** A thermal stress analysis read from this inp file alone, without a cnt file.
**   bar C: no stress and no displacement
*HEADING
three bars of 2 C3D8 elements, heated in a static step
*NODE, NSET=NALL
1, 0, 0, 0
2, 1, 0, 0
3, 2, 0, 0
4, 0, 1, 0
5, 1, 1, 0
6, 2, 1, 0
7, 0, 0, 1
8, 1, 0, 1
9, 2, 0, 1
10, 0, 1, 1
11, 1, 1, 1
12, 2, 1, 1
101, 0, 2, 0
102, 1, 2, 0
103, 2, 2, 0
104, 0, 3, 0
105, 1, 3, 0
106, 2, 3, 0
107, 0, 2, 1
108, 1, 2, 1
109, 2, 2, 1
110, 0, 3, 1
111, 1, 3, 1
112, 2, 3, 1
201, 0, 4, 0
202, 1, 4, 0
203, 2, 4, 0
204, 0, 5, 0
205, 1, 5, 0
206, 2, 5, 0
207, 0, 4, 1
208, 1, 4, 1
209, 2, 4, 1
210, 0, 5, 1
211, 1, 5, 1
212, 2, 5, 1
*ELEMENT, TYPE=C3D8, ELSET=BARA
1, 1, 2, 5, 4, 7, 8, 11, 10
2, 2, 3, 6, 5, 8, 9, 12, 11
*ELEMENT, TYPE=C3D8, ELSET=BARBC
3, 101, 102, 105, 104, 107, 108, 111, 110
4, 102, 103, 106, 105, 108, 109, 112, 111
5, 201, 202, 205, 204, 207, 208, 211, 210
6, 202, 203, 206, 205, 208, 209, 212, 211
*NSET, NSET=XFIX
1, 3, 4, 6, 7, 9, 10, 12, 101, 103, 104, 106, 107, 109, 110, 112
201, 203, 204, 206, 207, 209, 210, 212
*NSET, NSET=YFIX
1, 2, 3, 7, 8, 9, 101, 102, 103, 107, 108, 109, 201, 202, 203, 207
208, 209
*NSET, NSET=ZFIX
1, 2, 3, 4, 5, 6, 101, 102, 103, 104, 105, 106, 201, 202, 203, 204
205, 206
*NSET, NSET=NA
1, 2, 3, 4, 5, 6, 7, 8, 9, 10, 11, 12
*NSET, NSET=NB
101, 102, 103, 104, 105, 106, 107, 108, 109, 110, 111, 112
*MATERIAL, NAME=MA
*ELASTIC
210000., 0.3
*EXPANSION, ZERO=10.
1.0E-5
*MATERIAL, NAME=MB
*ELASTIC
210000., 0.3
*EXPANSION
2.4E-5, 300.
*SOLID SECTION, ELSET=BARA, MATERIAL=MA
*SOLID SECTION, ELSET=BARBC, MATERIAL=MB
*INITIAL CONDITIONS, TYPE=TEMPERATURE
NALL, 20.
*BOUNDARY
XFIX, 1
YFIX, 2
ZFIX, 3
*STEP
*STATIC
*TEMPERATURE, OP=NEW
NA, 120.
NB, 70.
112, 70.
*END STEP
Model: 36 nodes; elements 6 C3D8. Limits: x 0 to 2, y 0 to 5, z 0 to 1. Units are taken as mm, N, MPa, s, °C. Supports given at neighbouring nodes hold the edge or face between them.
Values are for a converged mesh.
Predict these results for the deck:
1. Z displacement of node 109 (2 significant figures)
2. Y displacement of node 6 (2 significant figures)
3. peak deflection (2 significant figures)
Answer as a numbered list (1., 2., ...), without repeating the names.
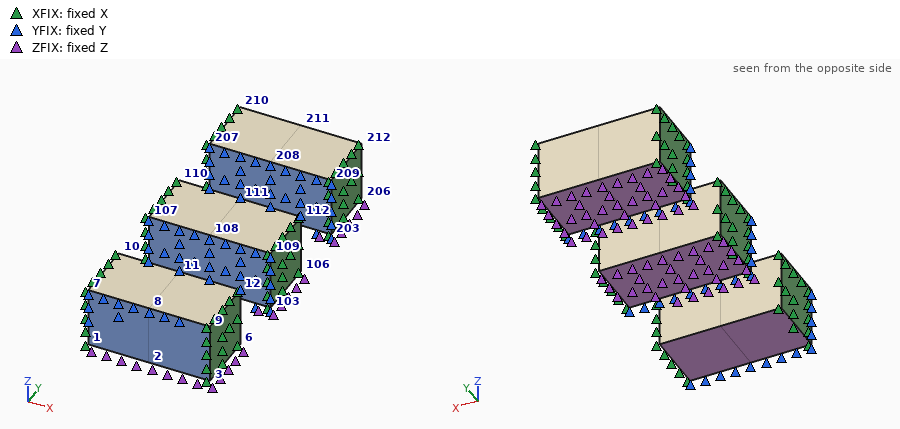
1. 0.0016 mm
2. 0.0013 mm
3. 0.0022 mm
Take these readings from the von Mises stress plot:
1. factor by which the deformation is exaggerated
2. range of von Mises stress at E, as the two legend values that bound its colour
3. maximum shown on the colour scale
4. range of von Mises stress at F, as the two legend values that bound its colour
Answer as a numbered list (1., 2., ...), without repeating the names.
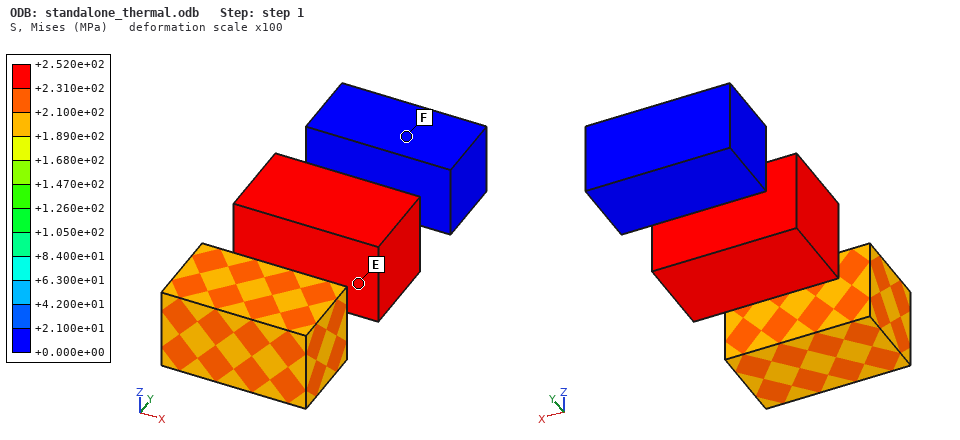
1. 100
2. +2.310e+02 to +2.520e+02 MPa
3. +2.520e+02 MPa
4. +0.000e+00 to +2.100e+01 MPa
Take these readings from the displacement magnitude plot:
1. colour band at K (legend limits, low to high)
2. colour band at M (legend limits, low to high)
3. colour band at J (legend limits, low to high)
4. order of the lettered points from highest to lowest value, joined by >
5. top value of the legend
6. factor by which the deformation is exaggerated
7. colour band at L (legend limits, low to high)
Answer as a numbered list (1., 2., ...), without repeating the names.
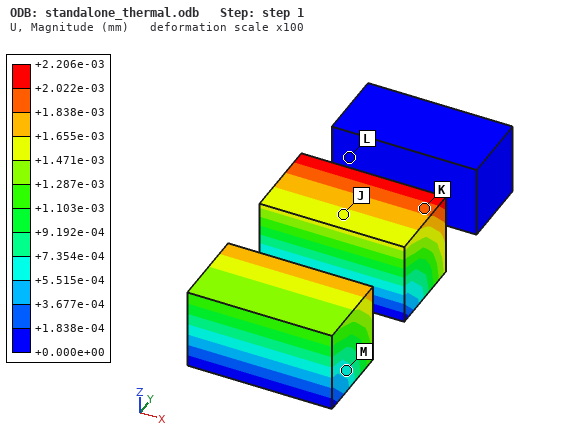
1. +1.838e-03 to +2.022e-03 mm
2. +5.515e-04 to +7.354e-04 mm
3. +1.471e-03 to +1.655e-03 mm
4. K > J > M > L
5. +2.206e-03 mm
6. 100
7. +0.000e+00 to +1.838e-04 mm
